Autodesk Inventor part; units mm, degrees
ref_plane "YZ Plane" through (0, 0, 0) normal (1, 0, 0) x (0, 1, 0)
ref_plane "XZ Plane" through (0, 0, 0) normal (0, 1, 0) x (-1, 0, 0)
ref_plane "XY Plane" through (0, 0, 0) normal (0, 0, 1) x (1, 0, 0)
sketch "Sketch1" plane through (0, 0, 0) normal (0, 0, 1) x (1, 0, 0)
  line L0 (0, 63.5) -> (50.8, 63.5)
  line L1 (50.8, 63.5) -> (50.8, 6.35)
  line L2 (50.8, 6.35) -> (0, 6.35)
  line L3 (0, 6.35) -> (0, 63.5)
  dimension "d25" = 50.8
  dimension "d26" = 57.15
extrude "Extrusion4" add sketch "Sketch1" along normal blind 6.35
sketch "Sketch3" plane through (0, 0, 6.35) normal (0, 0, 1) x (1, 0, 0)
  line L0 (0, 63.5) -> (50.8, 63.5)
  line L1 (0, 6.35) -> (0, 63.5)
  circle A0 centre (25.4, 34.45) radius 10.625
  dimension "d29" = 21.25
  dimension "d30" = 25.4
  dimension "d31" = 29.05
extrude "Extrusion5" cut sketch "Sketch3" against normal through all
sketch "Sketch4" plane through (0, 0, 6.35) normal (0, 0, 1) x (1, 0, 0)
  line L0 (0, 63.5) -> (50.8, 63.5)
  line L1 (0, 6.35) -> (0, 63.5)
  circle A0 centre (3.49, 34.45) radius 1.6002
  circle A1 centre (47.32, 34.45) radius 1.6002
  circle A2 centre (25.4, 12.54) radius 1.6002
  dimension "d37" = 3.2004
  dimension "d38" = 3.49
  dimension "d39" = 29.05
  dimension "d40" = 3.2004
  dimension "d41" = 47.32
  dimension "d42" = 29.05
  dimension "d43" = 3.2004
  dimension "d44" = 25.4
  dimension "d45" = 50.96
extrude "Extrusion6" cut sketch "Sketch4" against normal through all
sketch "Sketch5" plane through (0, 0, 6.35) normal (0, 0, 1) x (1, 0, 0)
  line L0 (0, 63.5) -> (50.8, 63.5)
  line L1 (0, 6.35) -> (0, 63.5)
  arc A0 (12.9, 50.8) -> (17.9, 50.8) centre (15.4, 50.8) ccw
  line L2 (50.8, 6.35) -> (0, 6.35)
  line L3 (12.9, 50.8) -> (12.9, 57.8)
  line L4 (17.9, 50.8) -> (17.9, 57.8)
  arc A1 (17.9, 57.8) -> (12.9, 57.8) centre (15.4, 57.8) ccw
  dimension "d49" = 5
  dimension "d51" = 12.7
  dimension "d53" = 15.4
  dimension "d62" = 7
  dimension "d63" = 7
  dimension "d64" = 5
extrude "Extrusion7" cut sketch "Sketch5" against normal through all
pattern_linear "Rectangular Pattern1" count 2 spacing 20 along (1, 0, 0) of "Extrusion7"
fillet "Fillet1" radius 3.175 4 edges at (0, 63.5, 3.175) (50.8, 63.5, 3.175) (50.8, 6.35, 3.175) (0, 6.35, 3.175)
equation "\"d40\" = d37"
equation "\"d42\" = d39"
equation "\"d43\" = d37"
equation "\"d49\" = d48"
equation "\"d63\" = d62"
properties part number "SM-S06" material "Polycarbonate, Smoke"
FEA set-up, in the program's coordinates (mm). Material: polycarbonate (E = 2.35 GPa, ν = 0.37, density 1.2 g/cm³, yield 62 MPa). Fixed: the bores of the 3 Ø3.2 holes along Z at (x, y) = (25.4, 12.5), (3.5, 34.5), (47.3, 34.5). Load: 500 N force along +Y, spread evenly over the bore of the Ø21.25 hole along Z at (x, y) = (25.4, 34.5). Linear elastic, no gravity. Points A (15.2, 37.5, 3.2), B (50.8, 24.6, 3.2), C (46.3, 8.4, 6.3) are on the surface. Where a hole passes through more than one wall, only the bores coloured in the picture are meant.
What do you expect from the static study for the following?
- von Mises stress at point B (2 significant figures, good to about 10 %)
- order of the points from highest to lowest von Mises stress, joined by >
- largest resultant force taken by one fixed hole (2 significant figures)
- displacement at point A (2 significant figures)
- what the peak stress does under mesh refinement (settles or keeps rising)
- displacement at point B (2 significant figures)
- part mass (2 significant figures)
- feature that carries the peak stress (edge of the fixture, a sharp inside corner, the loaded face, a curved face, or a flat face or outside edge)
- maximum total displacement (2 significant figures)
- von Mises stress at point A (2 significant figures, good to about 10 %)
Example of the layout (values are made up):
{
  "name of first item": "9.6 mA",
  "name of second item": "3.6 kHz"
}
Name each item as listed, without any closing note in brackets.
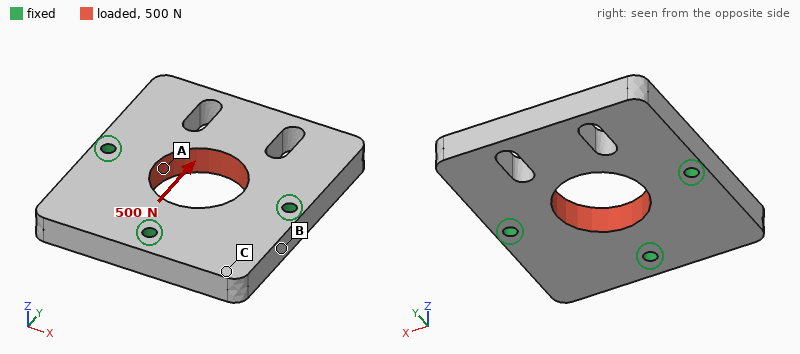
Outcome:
{
  "von Mises stress at point B": "1.4 MPa",
  "order of the points from highest to lowest von Mises stress, joined by >": "A > B > C",
  "largest resultant force taken by one fixed hole": "170 N",
  "displacement at point A": "20 µm",
  "what the peak stress does under mesh refinement": "keeps rising",
  "displacement at point B": "5.9 µm",
  "part mass": "18 g",
  "feature that carries the peak stress": "edge of the fixture",
  "maximum total displacement": "32 µm",
  "von Mises stress at point A": "2.8 MPa"
}
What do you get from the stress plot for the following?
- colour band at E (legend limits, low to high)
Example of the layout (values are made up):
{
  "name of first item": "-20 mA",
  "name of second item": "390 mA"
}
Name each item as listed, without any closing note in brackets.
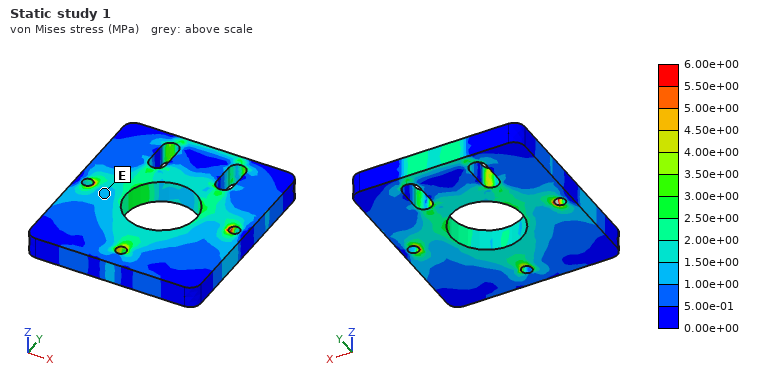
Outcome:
{
  "colour band at E": "1.00e+00 to 1.50e+00 MPa"
}
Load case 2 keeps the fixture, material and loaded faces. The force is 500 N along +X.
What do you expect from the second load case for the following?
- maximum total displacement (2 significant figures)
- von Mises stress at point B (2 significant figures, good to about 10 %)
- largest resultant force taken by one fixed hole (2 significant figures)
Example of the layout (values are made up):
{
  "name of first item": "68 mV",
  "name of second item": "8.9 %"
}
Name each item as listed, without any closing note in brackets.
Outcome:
{
  "maximum total displacement": "28 µm",
  "von Mises stress at point B": "1.0 MPa",
  "largest resultant force taken by one fixed hole": "200 N"
}
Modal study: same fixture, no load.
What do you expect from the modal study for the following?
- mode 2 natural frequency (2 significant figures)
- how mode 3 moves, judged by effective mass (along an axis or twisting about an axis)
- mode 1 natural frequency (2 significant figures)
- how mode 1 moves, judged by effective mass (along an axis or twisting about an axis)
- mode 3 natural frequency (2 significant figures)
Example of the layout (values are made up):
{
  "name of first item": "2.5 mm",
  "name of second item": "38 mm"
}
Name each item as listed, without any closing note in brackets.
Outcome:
{
  "mode 2 natural frequency": "2300 Hz",
  "how mode 3 moves, judged by effective mass": "twisting about Y",
  "mode 1 natural frequency": "1200 Hz",
  "how mode 1 moves, judged by effective mass": "along Z",
  "mode 3 natural frequency": "3400 Hz"
}
